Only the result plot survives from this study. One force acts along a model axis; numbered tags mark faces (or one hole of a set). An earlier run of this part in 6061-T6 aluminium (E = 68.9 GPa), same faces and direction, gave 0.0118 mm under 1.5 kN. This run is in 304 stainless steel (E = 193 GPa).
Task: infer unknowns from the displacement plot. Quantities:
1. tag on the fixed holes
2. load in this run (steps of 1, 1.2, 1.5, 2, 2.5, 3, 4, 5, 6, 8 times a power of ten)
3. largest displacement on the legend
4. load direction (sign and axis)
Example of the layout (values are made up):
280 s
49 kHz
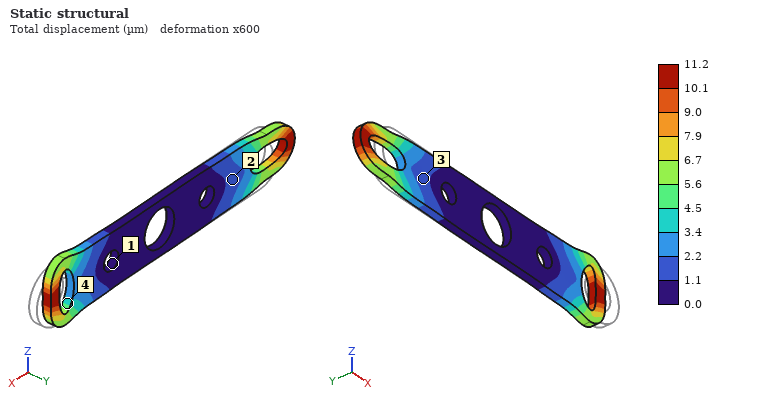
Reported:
1
4 kN
11.2 µm
-X
